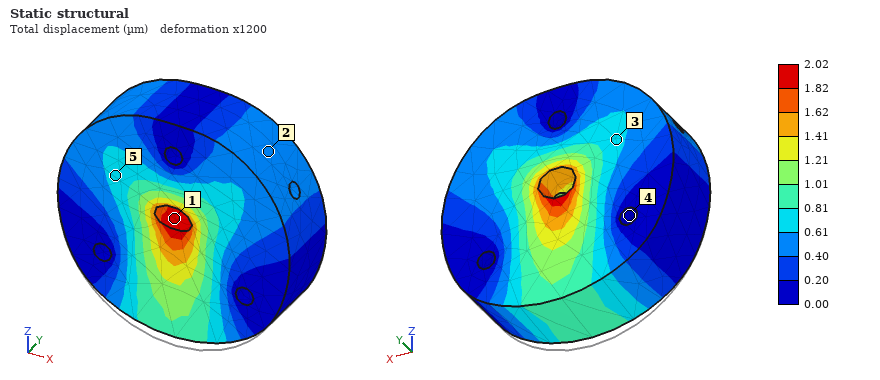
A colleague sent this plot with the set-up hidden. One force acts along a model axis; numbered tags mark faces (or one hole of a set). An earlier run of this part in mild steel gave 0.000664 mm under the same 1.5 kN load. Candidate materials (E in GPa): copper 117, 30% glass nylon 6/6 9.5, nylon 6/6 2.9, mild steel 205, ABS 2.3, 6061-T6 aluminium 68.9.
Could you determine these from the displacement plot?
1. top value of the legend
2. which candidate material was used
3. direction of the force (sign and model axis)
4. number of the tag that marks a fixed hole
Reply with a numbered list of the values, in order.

1. 2.02 µm
2. 6061-T6 aluminium
3. +Z
4. 4
